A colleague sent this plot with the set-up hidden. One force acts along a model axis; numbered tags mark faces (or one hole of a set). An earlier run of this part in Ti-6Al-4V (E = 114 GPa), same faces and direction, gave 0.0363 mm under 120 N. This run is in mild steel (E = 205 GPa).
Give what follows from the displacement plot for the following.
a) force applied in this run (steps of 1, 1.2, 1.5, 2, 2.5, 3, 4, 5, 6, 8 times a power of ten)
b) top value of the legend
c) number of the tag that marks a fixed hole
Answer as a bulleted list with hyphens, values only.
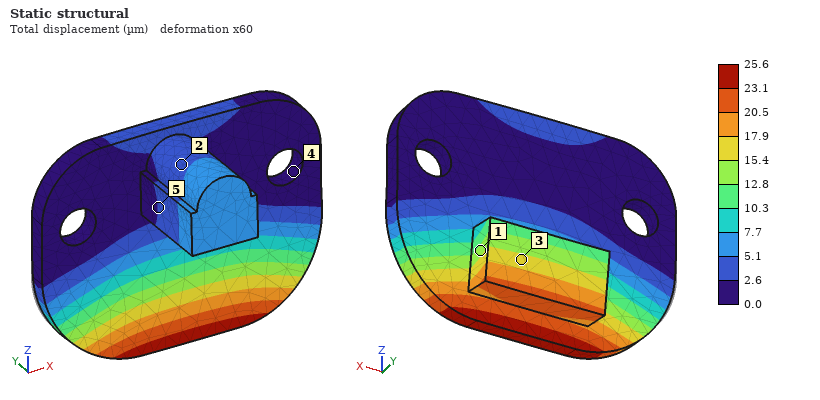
- 150 N
- 25.6 µm
- 4
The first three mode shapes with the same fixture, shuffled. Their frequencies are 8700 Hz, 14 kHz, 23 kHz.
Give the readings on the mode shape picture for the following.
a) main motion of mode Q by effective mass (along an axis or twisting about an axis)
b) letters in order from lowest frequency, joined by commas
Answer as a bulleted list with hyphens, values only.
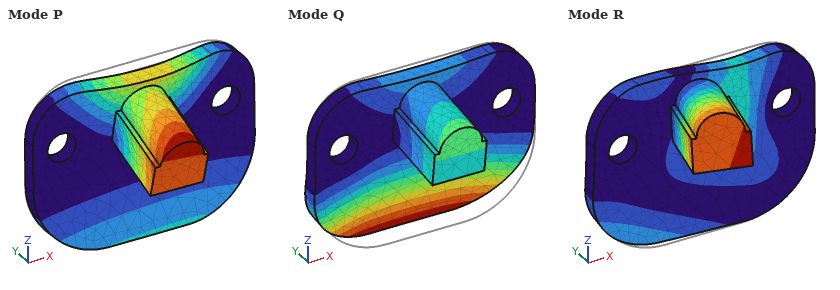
- along Y
- Q, P, R
